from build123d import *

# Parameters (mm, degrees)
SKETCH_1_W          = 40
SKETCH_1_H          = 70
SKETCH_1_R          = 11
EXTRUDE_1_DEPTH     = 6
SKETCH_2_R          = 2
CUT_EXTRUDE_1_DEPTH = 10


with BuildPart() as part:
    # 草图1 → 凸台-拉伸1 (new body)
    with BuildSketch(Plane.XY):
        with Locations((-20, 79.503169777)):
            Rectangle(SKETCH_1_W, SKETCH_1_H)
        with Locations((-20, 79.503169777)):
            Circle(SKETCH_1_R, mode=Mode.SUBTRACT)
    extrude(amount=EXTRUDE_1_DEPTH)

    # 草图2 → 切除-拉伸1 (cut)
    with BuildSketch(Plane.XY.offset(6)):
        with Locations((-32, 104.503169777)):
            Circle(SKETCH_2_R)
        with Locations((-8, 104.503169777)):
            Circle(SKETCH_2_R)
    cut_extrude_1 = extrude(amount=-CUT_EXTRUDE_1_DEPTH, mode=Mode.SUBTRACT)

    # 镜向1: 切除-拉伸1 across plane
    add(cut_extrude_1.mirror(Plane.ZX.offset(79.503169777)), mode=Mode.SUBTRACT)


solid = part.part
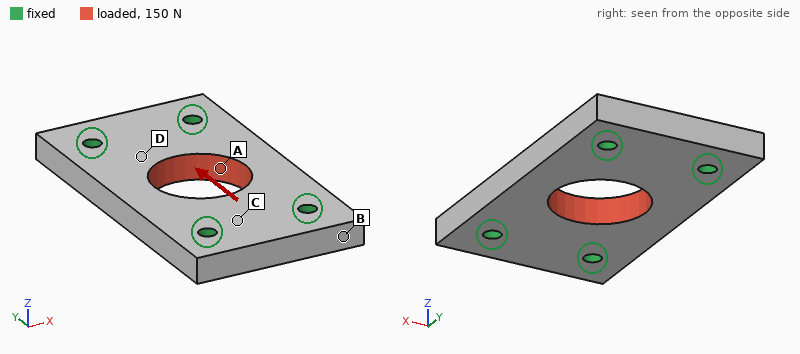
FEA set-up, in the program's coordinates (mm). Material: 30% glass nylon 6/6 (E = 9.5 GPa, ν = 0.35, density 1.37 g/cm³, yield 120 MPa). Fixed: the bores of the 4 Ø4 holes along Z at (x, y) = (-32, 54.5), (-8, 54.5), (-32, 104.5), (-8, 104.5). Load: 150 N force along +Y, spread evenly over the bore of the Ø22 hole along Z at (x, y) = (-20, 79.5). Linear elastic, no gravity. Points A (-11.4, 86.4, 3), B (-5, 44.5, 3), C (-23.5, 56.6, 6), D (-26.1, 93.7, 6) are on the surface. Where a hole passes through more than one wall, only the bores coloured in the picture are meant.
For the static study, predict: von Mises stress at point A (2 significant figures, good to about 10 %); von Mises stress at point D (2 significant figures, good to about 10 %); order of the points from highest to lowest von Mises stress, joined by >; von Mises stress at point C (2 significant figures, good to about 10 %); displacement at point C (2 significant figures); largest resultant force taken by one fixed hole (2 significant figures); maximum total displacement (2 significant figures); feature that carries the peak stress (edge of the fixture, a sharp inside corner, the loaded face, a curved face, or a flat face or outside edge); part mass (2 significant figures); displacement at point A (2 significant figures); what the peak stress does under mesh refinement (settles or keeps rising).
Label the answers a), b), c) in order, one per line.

a) 0.55 MPa
b) 0.39 MPa
c) A > D > C > B
d) 0.18 MPa
e) 0.39 µm
f) 38 N
g) 0.99 µm
h) edge of the fixture
i) 19 g
j) 0.86 µm
k) keeps rising
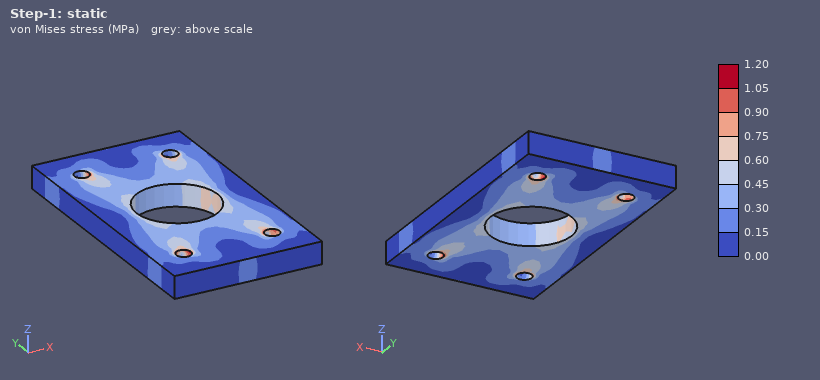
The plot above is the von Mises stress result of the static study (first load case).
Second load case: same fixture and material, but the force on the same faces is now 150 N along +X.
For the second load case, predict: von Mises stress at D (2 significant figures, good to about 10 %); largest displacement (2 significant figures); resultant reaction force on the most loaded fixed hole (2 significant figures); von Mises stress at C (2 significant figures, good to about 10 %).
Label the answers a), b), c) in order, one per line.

a) 0.73 MPa
b) 3.1 µm
c) 44 N
d) 0.57 MPa
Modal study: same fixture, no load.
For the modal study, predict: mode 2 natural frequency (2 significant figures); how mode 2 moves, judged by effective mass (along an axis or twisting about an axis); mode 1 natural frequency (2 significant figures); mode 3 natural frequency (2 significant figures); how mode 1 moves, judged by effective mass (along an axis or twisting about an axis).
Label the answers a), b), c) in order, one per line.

a) 7100 Hz
b) twisting about Y
c) 6400 Hz
d) 13 kHz
e) along Z
